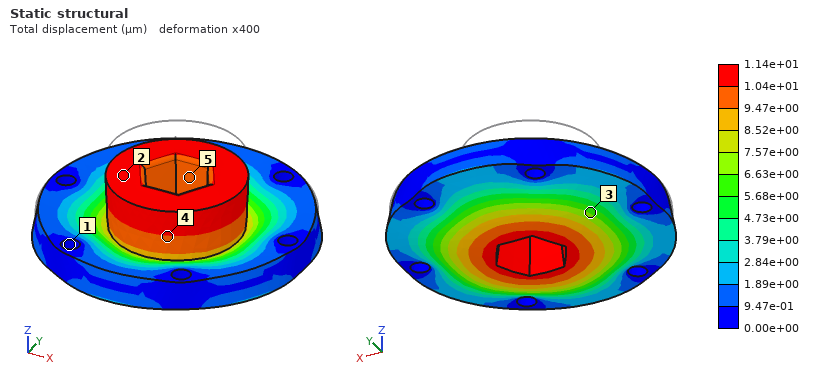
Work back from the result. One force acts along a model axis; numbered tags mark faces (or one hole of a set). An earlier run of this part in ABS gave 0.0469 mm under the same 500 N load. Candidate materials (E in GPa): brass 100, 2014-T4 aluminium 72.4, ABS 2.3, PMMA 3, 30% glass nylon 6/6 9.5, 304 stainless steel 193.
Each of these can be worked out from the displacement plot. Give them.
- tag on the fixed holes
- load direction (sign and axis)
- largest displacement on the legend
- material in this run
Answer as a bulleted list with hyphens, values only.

- 1
- -Z
- 1.14e+01 µm
- 30% glass nylon 6/6
